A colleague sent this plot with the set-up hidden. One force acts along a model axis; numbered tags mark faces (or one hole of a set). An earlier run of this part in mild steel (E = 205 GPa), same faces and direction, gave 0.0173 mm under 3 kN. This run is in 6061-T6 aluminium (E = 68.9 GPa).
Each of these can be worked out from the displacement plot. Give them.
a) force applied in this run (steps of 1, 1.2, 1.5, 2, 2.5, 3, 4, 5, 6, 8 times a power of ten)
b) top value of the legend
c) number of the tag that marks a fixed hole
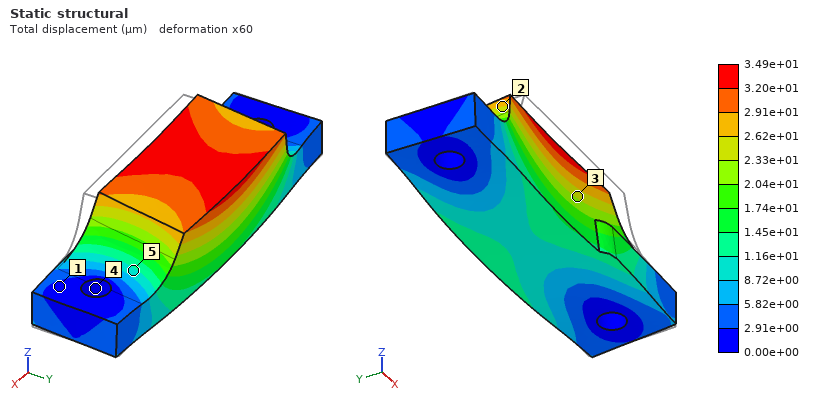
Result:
2 kN
3.49e+01 µm
4
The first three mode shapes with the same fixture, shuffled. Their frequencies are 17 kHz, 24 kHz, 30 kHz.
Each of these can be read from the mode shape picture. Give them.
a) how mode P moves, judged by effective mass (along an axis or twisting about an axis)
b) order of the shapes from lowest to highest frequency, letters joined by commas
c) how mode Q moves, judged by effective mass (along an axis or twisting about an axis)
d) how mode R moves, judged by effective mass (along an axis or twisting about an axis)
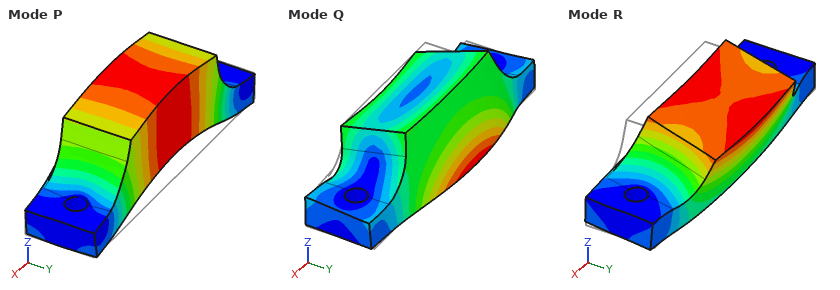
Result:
along Z
R, P, Q
along Y
along Y
